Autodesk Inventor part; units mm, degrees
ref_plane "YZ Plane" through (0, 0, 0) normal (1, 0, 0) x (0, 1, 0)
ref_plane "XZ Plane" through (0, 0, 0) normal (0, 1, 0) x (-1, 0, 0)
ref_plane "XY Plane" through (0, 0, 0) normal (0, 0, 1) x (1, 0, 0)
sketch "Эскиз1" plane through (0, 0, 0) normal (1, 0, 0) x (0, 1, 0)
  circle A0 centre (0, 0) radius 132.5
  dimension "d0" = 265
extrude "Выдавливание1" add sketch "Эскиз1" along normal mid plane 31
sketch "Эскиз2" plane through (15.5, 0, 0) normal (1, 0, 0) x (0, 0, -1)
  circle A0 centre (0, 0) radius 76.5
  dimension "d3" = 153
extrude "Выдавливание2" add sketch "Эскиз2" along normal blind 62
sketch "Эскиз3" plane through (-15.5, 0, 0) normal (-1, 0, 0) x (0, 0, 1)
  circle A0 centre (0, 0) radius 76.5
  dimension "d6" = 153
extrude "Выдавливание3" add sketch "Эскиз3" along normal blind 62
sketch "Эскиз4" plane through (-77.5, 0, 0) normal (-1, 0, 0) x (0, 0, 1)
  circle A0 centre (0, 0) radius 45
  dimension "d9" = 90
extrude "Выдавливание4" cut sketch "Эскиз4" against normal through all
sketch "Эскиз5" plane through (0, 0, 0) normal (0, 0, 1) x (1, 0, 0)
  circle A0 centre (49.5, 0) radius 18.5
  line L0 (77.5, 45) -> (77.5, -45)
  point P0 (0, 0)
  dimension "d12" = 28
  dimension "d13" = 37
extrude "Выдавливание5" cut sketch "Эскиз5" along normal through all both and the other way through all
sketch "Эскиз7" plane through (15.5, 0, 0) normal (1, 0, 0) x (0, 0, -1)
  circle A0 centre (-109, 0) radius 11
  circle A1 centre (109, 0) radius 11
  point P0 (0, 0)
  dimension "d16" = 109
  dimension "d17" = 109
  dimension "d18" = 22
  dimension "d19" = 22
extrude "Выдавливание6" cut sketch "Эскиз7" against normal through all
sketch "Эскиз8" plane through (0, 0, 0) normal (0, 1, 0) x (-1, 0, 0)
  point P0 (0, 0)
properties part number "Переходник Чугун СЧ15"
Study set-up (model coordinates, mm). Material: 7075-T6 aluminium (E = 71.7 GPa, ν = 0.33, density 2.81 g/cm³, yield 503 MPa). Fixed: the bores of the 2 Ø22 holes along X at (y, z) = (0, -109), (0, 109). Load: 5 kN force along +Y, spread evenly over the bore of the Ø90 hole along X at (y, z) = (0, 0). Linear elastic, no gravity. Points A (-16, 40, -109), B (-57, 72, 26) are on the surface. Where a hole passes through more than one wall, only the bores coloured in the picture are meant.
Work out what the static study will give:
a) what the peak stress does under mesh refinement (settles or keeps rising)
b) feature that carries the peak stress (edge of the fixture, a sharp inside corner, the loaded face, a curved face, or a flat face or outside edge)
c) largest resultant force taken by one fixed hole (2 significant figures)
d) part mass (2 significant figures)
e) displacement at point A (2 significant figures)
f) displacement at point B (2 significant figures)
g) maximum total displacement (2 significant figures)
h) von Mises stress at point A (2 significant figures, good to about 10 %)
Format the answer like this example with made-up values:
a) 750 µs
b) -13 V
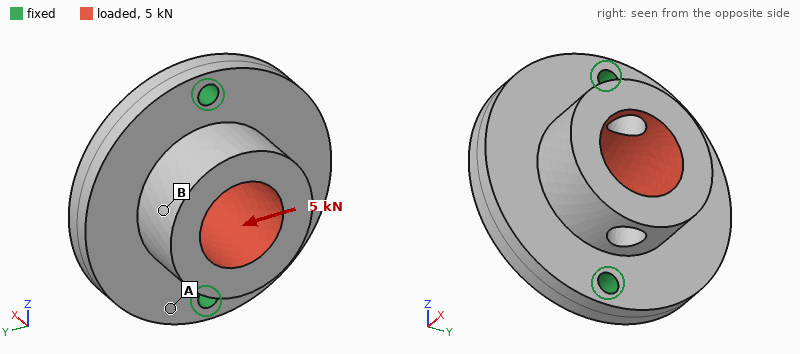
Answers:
a) keeps rising
b) edge of the fixture
c) 2.5 kN
d) 8.2 kg
e) 0.48 µm
f) 2.2 µm
g) 2.6 µm
h) 0.69 MPa
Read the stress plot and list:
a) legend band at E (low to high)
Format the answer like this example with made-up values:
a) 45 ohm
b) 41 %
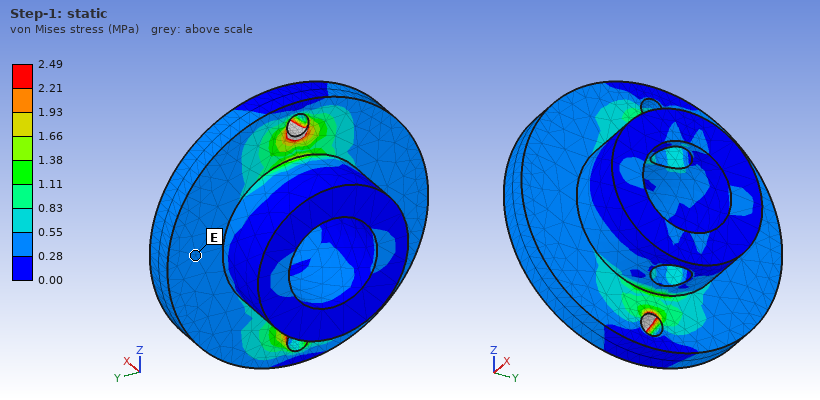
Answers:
a) 0.28 to 0.55 MPa
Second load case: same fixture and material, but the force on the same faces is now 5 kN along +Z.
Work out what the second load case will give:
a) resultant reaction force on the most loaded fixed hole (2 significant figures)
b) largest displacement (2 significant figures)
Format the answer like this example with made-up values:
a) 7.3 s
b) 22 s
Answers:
a) 2.5 kN
b) 1.5 µm
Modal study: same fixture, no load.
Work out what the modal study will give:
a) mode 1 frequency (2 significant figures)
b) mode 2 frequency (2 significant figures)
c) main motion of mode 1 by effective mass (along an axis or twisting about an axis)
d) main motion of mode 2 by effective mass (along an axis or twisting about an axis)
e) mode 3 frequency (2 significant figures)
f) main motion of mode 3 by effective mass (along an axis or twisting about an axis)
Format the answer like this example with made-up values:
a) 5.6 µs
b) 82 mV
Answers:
a) 960 Hz
b) 2000 Hz
c) twisting about Z
d) along X
e) 3500 Hz
f) twisting about Y
